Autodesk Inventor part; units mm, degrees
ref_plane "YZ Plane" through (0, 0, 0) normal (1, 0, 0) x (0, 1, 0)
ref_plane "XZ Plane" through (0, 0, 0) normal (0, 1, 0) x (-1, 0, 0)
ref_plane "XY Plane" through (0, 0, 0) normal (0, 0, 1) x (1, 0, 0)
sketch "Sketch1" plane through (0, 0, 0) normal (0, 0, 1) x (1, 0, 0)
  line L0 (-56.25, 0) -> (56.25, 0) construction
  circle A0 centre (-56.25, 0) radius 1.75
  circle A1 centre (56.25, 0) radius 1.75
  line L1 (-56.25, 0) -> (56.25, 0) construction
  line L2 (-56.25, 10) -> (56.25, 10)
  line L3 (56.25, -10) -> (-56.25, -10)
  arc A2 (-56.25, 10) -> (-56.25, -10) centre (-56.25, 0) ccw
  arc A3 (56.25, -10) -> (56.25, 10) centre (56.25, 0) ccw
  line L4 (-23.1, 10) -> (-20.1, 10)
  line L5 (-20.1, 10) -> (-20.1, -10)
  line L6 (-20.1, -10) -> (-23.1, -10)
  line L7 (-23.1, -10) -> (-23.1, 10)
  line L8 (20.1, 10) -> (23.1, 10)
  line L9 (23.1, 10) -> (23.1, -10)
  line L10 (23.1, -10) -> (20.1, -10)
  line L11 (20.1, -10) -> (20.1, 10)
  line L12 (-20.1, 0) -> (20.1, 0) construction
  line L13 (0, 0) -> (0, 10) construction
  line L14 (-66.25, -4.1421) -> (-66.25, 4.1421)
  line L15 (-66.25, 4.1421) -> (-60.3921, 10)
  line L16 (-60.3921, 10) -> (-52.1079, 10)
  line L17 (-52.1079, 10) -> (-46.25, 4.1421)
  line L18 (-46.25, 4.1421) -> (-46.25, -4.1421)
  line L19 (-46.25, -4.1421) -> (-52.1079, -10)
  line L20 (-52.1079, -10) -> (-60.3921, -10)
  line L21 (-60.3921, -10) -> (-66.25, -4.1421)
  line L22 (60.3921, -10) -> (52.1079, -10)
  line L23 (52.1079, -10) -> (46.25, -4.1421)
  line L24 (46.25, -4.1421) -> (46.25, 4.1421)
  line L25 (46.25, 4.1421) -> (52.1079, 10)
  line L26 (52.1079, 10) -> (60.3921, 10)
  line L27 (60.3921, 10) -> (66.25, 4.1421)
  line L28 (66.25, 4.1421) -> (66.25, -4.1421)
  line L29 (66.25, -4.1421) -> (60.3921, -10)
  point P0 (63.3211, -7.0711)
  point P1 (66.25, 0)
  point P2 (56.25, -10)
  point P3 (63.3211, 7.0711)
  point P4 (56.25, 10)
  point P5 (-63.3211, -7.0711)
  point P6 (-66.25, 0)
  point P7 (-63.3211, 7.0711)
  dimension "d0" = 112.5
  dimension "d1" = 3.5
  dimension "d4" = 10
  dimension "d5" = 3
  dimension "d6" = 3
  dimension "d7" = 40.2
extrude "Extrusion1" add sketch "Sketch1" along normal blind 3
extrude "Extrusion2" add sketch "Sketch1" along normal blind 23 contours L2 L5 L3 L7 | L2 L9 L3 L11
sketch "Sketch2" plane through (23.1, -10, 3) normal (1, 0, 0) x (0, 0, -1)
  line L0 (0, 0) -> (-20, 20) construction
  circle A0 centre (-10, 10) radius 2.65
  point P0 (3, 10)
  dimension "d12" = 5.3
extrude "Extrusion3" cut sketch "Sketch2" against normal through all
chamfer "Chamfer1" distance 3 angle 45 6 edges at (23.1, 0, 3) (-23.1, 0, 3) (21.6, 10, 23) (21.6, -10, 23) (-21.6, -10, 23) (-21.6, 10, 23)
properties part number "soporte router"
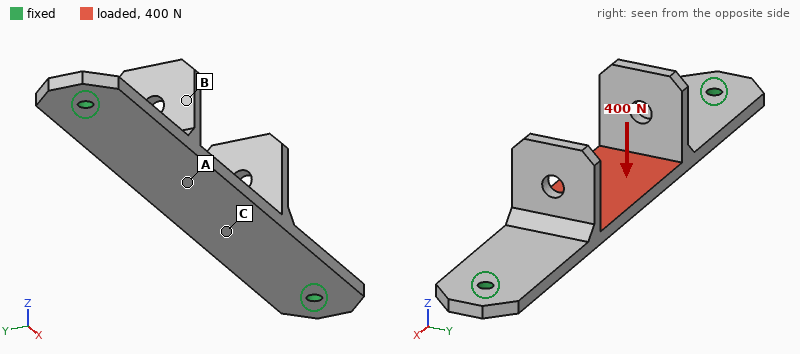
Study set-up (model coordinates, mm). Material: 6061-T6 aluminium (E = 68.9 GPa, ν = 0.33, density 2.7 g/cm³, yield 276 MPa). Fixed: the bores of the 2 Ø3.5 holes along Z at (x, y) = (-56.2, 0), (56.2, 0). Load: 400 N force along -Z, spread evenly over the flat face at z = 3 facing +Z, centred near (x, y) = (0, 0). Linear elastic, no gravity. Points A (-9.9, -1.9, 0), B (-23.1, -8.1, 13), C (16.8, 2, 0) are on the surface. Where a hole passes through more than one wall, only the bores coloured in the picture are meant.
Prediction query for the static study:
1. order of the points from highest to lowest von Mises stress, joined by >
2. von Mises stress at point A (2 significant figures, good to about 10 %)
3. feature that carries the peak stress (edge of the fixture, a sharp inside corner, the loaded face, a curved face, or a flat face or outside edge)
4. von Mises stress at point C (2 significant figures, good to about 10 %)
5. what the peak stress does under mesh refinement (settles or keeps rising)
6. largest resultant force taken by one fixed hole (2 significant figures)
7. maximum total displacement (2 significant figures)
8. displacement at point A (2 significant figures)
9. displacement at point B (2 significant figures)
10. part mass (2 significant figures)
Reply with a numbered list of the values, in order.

1. A > C > B
2. 110 MPa
3. edge of the fixture
4. 78 MPa
5. keeps rising
6. 200 N
7. 0.86 mm
8. 0.78 mm
9. 0.60 mm
10. 27 g
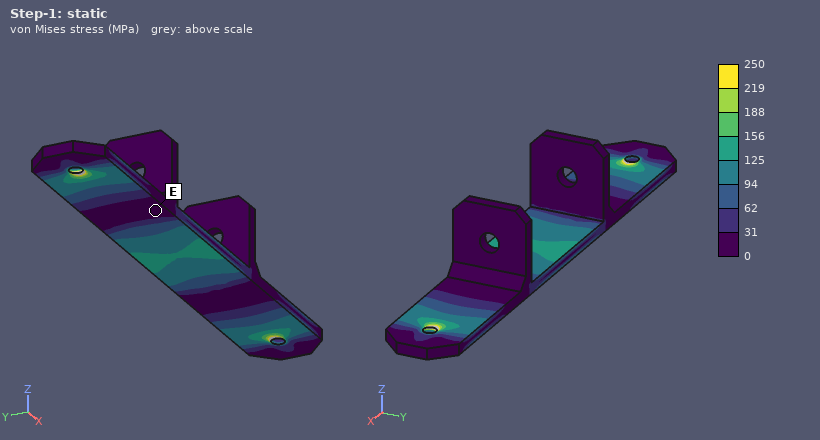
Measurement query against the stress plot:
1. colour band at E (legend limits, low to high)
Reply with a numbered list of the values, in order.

1. 0 to 31 MPa
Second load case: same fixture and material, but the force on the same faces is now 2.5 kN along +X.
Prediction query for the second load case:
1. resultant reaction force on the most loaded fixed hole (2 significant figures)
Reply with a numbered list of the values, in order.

1. 1.3 kN
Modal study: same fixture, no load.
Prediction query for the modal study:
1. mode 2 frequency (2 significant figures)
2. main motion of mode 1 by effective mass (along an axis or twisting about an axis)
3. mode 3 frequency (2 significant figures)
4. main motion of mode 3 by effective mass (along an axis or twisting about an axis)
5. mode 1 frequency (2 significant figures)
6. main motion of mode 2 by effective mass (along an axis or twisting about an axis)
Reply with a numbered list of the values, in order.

1. 2100 Hz
2. along Z
3. 2700 Hz
4. twisting about Y
5. 1000 Hz
6. along Y
